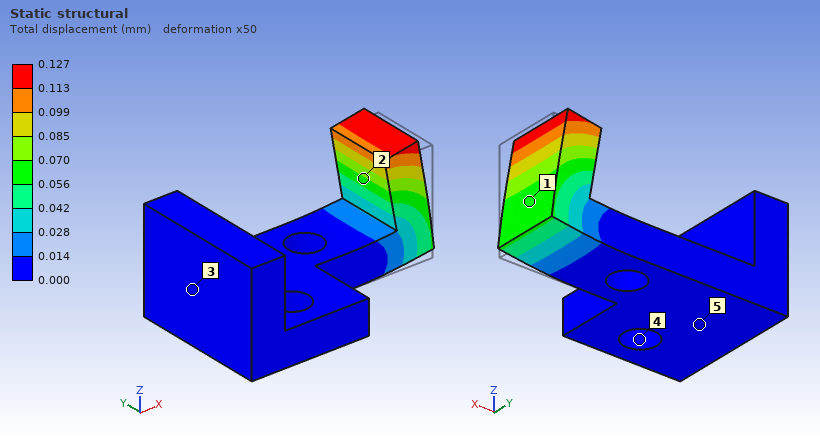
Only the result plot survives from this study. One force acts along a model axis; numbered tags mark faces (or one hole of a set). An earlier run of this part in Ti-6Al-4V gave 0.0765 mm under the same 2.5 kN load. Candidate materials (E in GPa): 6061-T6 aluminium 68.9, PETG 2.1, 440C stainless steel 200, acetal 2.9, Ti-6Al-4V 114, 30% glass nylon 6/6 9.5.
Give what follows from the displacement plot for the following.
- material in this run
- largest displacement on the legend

6061-T6 aluminium
0.127 mm
